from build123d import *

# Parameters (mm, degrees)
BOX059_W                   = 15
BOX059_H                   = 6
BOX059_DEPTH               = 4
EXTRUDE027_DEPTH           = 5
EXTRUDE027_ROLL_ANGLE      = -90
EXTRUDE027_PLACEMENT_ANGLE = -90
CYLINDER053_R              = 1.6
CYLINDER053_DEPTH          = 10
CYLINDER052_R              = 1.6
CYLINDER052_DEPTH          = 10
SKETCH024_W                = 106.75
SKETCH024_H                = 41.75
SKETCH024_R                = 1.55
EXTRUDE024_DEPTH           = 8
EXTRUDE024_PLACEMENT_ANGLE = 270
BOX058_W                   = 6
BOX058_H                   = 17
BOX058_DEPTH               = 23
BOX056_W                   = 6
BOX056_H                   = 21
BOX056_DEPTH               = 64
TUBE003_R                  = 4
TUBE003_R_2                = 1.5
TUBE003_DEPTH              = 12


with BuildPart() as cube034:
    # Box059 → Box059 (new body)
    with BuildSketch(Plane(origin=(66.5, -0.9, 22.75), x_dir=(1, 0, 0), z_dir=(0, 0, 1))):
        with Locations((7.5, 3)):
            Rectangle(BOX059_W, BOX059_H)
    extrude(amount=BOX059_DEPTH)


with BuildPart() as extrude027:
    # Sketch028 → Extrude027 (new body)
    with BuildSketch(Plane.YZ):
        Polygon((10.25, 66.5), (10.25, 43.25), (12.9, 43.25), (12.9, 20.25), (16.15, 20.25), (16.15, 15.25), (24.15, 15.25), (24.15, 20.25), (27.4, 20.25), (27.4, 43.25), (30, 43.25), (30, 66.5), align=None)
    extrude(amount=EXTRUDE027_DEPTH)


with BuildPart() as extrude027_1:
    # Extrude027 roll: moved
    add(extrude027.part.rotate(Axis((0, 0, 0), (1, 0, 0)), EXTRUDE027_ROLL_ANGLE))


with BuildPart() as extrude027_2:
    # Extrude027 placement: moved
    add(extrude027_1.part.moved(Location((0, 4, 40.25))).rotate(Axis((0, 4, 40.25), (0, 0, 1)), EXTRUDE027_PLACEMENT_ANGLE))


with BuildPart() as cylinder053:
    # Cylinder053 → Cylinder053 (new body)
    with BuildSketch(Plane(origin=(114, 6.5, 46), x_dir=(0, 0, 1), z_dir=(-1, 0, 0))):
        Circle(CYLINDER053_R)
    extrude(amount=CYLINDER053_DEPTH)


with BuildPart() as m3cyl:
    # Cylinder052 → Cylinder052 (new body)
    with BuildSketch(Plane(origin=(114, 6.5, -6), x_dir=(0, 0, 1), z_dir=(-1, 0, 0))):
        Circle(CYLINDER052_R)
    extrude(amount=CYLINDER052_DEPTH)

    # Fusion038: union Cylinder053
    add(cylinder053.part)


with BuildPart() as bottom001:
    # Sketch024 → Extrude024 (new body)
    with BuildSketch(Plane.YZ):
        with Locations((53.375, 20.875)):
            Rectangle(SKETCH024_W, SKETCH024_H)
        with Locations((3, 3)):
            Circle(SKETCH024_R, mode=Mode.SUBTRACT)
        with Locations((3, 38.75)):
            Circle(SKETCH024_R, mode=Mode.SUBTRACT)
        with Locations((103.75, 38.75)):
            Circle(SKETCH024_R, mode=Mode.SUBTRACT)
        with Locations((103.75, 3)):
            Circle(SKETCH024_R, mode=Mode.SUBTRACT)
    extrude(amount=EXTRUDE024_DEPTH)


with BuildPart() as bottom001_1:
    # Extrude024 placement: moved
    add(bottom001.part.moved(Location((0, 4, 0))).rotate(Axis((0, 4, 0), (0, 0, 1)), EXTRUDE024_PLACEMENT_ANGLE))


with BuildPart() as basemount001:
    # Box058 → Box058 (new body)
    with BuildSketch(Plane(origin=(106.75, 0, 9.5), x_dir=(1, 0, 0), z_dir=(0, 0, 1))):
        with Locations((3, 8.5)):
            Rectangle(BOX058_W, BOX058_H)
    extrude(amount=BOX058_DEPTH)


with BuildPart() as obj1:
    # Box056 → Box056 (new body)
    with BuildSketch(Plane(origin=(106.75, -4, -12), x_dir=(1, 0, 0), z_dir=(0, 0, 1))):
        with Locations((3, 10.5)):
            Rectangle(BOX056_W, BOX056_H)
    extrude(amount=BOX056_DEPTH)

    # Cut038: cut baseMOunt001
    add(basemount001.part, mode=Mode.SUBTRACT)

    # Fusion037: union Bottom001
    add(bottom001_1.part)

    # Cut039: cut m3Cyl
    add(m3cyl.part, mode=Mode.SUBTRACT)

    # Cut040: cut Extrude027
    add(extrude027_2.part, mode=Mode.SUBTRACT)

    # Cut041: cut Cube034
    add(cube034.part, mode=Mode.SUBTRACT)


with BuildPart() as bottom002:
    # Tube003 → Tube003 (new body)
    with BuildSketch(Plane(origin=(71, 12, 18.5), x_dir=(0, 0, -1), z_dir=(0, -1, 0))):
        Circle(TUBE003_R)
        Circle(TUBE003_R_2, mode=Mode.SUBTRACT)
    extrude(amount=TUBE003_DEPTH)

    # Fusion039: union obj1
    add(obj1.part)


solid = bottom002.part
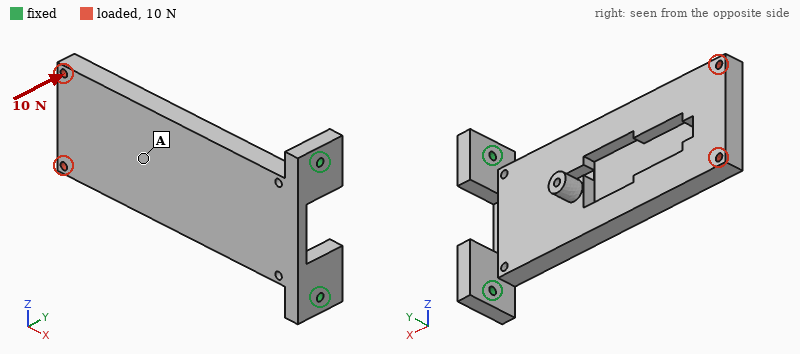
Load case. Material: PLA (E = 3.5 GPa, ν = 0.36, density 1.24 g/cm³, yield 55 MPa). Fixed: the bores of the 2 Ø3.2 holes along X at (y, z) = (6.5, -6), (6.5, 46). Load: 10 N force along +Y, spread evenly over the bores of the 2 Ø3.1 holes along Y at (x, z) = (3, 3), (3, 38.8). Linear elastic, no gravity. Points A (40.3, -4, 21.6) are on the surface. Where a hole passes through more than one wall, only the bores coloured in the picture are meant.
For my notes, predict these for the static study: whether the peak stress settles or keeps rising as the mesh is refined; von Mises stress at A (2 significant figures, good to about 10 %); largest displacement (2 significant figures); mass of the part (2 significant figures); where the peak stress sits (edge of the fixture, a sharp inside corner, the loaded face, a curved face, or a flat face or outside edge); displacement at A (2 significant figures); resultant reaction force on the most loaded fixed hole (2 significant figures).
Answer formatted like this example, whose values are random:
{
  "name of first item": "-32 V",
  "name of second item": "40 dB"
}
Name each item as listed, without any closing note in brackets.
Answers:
{
  "whether the peak stress settles or keeps rising as the mesh is refined": "keeps rising",
  "von Mises stress at A": "0.93 MPa",
  "largest displacement": "1.4 mm",
  "mass of the part": "46 g",
  "where the peak stress sits": "edge of the fixture",
  "displacement at A": "0.78 mm",
  "resultant reaction force on the most loaded fixed hole": "7.2 N"
}
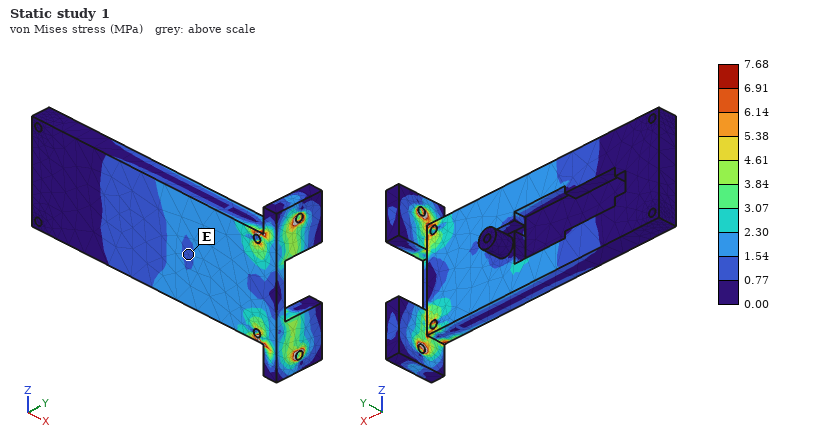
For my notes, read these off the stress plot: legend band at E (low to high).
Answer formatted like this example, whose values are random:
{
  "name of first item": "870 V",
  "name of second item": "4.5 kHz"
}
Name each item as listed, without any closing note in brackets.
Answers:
{
  "legend band at E": "0.77 to 1.54 MPa"
}
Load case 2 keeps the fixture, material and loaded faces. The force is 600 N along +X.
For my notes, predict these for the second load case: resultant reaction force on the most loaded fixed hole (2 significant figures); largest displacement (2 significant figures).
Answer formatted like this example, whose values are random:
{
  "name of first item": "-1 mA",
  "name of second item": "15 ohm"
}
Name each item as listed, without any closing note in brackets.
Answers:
{
  "resultant reaction force on the most loaded fixed hole": "320 N",
  "largest displacement": "1.1 mm"
}
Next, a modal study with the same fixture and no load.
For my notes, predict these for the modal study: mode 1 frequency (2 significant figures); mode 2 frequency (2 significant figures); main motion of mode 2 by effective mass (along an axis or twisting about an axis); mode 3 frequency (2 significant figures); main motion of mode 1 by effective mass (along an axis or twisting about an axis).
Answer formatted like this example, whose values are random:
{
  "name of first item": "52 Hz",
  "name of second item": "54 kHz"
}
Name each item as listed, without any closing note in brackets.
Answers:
{
  "mode 1 frequency": "120 Hz",
  "mode 2 frequency": "530 Hz",
  "main motion of mode 2 by effective mass": "along Z",
  "mode 3 frequency": "760 Hz",
  "main motion of mode 1 by effective mass": "along Y"
}
